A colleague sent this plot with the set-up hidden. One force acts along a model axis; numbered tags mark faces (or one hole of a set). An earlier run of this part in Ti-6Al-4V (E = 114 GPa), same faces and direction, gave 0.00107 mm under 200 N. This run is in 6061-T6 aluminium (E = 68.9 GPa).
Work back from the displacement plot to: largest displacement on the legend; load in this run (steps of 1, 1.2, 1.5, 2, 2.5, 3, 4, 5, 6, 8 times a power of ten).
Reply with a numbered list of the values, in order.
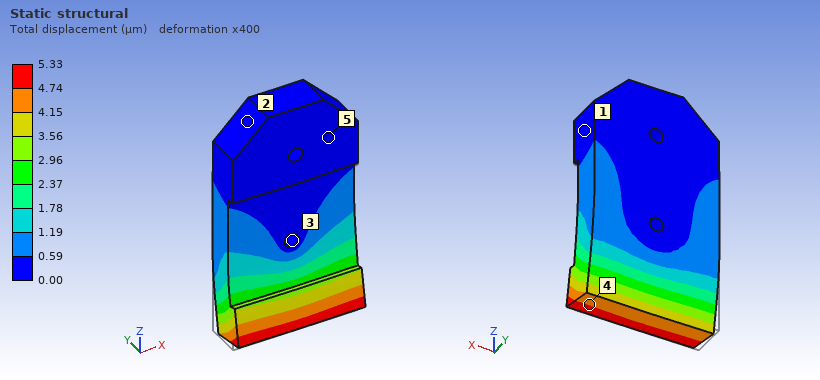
1. 5.33 µm
2. 600 N
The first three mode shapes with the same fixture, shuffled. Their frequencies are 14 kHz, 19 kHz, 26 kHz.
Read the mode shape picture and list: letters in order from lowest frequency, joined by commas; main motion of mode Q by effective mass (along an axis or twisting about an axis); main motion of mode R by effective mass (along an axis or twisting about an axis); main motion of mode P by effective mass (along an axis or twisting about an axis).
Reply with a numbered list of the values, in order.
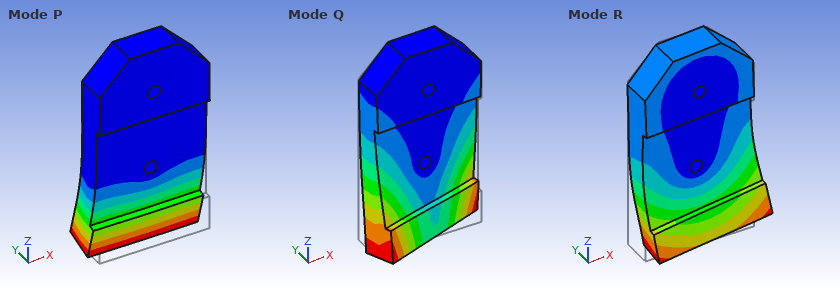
1. P, Q, R
2. twisting about Z
3. along X
4. along Y
